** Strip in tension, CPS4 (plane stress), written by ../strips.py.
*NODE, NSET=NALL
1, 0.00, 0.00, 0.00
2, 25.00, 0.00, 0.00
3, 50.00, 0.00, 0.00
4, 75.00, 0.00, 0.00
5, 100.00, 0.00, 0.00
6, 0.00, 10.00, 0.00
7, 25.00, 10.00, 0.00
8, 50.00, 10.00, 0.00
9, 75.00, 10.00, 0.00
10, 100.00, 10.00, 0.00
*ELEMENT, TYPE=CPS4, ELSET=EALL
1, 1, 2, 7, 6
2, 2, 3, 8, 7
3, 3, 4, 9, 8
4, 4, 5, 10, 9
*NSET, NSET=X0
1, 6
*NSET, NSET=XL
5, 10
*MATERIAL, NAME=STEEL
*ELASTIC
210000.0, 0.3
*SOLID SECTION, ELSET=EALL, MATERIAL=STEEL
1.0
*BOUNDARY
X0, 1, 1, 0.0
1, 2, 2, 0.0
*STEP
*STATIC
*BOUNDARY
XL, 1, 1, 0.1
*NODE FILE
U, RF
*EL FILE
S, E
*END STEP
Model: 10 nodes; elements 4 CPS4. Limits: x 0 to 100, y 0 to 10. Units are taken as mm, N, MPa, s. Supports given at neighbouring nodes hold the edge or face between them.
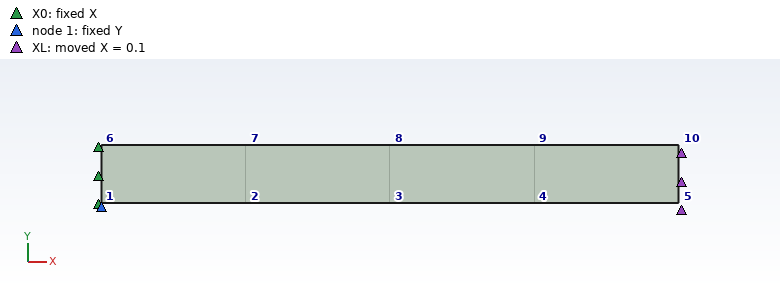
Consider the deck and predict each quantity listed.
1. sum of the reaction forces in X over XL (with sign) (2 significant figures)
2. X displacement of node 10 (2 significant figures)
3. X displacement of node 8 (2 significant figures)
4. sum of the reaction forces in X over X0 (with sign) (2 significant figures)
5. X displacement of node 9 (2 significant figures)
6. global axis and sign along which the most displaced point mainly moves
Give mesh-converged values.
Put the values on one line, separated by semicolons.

2100 N; 0.10 mm; 0.050 mm; -2100 N; 0.075 mm; +X
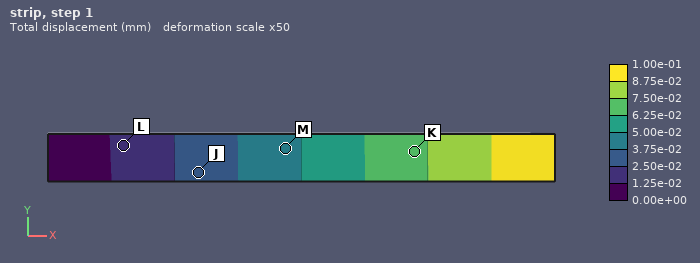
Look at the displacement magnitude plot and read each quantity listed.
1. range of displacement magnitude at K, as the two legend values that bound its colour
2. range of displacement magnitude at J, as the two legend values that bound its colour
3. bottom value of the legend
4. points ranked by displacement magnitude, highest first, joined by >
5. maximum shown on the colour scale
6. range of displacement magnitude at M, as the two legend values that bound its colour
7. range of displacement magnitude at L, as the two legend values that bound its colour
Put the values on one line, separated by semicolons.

6.25e-02 to 7.50e-02 mm; 2.50e-02 to 3.75e-02 mm; 0.00e+00 mm; K > M > J > L; 1.00e-01 mm; 3.75e-02 to 5.00e-02 mm; 1.25e-02 to 2.50e-02 mm
